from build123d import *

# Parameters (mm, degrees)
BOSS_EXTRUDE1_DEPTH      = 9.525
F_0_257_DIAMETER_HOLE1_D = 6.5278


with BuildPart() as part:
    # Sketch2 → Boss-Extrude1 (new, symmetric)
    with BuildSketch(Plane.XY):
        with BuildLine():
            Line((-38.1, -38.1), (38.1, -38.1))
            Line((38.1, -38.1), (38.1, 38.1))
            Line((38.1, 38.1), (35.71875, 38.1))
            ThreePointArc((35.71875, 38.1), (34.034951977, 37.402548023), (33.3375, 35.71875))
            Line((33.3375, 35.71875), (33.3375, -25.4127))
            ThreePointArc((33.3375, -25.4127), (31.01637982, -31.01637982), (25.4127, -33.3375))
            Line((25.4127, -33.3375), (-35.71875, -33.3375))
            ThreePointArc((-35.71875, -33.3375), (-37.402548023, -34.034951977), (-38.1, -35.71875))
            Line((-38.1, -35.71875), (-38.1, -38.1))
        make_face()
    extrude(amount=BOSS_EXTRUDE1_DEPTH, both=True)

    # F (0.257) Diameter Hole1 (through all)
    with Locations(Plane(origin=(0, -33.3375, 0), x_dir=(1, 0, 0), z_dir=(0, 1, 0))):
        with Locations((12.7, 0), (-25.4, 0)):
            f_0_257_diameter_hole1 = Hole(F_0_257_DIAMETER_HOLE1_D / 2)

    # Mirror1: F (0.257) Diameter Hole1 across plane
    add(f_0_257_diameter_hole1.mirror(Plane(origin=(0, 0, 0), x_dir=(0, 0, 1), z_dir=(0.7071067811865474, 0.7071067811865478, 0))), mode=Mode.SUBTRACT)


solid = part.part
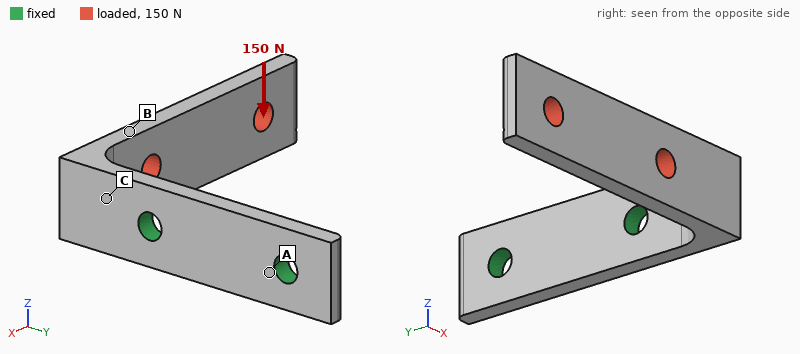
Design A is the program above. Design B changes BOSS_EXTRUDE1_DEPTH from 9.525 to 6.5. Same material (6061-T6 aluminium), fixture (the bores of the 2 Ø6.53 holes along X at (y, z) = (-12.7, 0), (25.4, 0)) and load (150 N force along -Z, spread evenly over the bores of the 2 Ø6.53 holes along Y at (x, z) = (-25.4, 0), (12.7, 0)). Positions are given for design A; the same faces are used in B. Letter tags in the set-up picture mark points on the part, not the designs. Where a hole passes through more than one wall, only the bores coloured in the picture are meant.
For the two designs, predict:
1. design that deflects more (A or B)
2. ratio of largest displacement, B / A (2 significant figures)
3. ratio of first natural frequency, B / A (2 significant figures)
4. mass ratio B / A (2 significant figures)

B
1.8
1.0
0.67
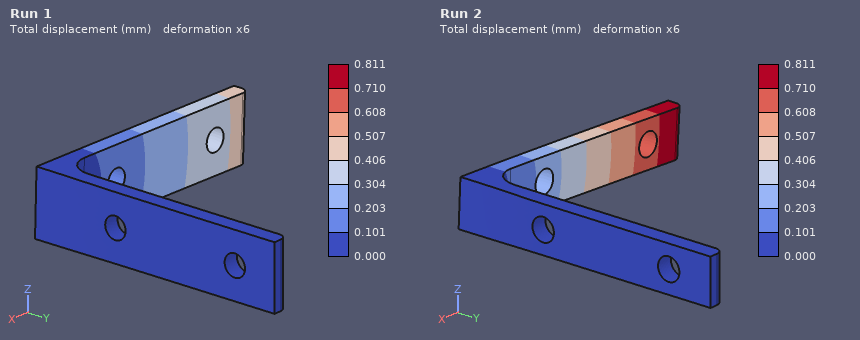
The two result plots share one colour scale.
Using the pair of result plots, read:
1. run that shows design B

Run 2
